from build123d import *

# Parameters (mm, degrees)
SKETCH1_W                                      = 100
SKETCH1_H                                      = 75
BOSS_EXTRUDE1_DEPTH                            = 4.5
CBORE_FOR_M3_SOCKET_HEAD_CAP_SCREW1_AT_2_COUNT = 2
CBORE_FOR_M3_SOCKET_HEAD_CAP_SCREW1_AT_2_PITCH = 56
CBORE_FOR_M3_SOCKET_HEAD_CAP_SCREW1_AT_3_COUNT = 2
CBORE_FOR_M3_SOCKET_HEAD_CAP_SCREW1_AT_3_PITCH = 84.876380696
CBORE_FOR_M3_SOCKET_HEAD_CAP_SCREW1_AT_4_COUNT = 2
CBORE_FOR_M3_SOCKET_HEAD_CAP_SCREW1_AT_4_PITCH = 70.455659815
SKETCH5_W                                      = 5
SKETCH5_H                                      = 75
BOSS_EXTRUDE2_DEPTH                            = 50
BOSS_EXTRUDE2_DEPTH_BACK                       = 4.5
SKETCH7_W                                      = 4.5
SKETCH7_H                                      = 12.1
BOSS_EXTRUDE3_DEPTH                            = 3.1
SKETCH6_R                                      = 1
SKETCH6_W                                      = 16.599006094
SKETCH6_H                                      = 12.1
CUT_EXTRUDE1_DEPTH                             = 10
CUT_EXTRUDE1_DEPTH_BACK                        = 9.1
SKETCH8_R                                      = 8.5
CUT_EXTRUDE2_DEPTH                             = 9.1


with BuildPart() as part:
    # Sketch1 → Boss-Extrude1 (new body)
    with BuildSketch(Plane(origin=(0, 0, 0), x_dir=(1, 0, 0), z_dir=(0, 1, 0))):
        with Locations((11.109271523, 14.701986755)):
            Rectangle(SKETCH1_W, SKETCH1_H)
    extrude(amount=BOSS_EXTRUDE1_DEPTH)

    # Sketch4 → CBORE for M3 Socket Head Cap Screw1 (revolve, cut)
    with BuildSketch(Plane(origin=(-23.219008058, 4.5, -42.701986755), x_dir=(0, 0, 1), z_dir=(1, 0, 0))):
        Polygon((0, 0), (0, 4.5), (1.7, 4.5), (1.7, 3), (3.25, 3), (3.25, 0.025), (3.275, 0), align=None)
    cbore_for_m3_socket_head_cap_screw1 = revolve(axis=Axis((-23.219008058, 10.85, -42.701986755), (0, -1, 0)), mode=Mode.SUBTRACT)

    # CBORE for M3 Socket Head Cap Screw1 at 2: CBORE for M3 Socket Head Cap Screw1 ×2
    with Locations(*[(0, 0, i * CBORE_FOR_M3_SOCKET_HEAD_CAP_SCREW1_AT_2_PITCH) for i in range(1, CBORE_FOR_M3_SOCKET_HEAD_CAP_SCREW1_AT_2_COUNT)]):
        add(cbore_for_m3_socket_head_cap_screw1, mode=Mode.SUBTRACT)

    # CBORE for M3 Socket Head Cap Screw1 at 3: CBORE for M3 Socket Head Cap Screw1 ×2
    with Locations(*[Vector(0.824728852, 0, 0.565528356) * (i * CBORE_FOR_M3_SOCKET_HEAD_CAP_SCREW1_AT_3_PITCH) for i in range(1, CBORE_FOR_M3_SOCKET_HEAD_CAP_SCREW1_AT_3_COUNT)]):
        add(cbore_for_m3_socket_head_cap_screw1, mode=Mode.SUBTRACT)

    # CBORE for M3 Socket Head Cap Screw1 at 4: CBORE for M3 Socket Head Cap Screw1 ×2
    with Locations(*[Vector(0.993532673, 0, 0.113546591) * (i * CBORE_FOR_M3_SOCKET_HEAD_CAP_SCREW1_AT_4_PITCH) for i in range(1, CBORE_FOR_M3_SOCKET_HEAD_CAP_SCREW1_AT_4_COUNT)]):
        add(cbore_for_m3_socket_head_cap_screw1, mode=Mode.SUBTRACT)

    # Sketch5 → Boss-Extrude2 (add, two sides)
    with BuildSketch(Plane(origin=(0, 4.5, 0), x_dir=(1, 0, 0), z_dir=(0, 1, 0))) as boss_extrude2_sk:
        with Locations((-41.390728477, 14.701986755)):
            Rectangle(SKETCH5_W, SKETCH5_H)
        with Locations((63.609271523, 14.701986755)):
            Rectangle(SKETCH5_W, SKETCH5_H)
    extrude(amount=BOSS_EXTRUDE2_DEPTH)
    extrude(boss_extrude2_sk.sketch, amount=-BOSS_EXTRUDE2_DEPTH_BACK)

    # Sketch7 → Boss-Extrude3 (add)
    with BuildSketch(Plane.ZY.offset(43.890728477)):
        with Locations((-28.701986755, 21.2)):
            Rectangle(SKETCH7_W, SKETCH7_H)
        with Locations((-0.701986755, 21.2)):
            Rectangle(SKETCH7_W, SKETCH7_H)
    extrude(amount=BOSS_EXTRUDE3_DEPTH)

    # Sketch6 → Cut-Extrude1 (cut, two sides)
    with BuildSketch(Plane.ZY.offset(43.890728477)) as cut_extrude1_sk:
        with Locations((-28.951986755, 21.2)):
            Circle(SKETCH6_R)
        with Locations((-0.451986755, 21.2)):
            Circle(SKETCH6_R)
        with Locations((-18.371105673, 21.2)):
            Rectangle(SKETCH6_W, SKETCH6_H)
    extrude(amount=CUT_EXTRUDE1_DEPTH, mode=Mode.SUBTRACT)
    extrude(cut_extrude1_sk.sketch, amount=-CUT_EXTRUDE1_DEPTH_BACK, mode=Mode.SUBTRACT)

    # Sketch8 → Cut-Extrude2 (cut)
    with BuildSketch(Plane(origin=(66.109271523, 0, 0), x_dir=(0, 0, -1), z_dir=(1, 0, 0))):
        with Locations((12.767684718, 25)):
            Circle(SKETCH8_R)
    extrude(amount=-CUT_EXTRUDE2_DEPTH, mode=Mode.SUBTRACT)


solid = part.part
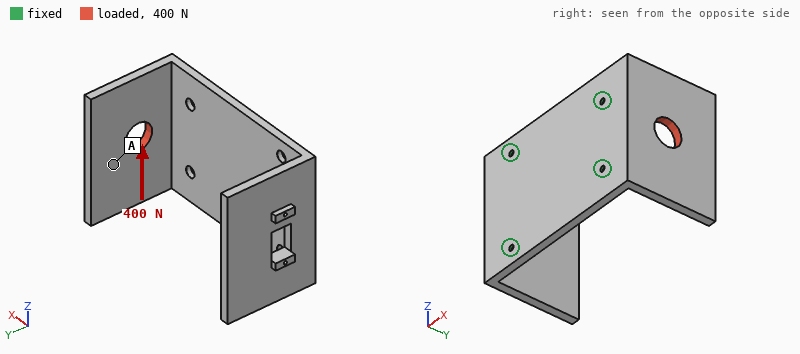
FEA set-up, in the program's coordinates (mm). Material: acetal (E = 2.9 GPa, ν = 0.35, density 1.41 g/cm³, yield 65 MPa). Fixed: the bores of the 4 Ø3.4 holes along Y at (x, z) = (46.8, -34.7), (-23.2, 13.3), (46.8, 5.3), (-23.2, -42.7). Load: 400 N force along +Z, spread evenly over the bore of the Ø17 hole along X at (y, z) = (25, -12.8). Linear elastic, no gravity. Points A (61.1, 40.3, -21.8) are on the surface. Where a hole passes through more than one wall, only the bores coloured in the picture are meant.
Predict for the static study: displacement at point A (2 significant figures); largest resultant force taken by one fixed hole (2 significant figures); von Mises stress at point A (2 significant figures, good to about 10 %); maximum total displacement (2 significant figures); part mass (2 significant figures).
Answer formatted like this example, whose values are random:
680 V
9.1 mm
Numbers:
0.91 mm
390 N
2.0 MPa
1.5 mm
100 g
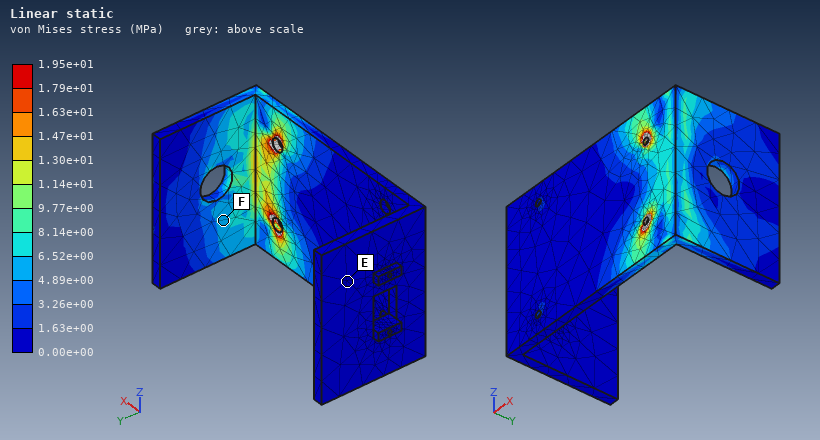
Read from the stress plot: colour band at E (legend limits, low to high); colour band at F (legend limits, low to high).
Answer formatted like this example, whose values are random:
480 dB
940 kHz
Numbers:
0.00e+00 to 1.63e+00 MPa
4.89e+00 to 6.52e+00 MPa
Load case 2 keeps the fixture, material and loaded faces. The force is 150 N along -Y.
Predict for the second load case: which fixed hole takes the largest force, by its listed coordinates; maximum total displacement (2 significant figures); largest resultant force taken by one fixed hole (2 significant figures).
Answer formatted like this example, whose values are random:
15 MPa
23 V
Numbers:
(46.8, 5.3)
1.6 mm
150 N
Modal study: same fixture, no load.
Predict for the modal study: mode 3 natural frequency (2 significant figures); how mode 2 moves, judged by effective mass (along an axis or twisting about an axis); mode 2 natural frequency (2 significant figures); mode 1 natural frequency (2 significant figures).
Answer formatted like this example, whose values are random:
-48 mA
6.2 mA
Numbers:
470 Hz
along X
210 Hz
200 Hz
